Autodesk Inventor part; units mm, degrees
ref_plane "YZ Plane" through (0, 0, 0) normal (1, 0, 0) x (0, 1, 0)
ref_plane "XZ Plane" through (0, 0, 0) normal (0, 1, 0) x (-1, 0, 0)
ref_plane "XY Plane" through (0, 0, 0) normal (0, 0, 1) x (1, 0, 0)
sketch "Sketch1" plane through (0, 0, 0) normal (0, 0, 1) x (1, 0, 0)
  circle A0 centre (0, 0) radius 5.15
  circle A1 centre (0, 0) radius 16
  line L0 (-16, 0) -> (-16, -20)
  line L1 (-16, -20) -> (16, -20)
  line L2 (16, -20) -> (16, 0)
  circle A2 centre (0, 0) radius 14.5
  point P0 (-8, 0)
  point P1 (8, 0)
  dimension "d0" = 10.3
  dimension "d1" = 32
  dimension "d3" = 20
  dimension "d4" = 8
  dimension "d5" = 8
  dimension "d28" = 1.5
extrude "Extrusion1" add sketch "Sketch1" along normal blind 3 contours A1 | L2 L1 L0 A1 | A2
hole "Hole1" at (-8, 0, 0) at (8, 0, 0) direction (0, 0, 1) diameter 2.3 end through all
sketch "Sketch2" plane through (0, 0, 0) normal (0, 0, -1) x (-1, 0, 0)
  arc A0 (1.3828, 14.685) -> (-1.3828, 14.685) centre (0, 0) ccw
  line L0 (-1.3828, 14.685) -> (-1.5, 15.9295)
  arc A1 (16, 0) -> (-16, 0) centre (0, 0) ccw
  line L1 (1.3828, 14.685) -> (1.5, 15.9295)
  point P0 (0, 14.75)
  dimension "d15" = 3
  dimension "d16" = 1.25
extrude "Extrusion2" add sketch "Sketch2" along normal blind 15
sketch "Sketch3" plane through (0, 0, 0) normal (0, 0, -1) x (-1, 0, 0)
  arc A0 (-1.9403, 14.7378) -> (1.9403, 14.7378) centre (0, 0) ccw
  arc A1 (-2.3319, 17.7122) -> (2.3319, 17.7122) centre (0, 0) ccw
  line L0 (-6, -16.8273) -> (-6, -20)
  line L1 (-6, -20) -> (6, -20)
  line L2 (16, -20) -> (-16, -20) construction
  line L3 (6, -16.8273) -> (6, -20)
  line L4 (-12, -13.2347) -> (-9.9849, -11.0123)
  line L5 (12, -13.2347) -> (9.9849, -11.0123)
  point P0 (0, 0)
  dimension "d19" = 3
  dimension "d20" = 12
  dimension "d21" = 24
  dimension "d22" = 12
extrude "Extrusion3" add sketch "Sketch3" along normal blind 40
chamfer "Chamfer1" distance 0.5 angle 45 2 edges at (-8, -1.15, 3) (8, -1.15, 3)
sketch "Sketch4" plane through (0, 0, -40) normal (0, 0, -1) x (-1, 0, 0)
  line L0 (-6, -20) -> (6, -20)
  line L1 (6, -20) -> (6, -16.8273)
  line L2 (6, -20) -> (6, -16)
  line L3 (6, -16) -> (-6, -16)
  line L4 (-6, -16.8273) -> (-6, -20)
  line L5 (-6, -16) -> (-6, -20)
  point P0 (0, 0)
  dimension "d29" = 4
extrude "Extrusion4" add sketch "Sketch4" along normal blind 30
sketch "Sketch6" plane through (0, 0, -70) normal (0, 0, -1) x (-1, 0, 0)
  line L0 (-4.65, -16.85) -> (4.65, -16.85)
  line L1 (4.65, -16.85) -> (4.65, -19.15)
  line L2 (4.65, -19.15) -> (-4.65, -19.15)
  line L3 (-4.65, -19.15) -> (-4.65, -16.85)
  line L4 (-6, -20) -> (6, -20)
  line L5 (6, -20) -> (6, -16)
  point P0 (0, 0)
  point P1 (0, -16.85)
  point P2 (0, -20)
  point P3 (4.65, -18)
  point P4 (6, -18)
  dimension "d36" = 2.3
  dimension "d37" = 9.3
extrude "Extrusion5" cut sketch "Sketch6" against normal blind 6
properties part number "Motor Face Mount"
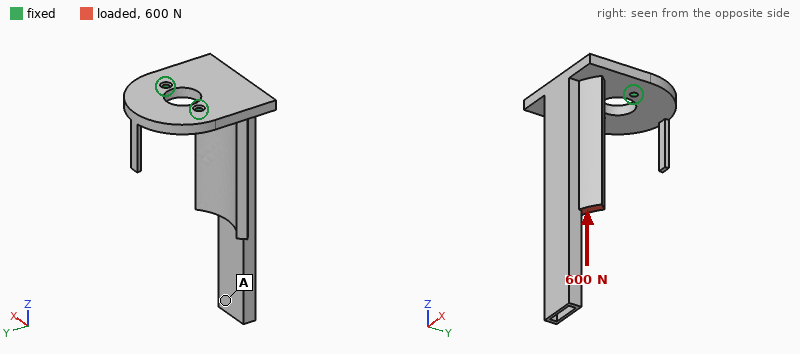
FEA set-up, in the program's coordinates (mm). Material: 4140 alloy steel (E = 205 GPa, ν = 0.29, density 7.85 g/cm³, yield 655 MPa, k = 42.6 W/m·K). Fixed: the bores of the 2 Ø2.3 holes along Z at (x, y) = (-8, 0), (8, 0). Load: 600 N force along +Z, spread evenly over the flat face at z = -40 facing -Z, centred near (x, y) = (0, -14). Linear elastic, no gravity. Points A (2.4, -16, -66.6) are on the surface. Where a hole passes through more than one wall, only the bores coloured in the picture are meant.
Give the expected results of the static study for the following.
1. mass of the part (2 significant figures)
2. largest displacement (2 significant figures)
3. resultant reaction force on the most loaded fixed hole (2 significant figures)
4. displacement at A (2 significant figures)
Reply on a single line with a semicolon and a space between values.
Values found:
65 g; 0.43 mm; 300 N; 0.41 mm
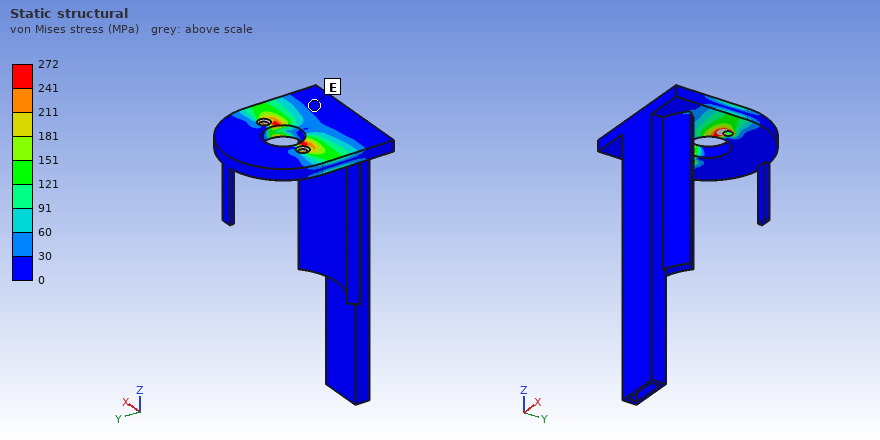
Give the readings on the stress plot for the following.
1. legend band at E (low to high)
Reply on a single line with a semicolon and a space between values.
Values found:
0 to 30 MPa
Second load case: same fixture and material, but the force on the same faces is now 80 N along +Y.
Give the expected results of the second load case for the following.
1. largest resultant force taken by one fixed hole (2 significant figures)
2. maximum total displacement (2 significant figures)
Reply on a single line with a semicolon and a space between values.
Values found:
42 N; 0.36 mm
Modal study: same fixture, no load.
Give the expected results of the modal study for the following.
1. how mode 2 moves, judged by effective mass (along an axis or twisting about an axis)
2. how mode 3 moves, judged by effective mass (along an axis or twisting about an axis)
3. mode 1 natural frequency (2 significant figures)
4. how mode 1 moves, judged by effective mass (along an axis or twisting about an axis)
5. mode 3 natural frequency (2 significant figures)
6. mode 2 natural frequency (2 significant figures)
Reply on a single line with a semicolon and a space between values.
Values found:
along X; along Z; 560 Hz; along Y; 3300 Hz; 1300 Hz
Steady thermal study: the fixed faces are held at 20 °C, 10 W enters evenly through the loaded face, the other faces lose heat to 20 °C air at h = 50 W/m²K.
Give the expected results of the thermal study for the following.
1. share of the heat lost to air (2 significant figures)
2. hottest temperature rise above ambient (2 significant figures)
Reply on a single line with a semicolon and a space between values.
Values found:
72 %; 74 K
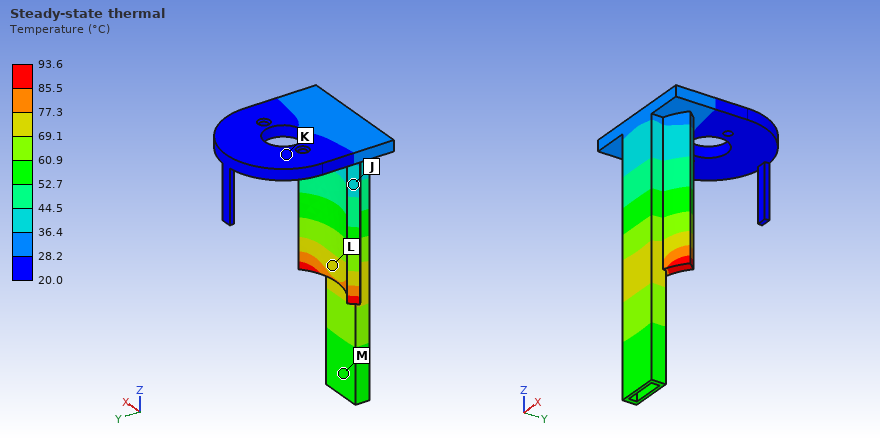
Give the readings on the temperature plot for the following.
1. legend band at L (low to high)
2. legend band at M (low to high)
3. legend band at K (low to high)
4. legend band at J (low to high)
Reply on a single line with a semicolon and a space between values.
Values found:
69.1 to 77.3 °C; 52.7 to 60.9 °C; 20.0 to 28.2 °C; 36.4 to 44.5 °C
